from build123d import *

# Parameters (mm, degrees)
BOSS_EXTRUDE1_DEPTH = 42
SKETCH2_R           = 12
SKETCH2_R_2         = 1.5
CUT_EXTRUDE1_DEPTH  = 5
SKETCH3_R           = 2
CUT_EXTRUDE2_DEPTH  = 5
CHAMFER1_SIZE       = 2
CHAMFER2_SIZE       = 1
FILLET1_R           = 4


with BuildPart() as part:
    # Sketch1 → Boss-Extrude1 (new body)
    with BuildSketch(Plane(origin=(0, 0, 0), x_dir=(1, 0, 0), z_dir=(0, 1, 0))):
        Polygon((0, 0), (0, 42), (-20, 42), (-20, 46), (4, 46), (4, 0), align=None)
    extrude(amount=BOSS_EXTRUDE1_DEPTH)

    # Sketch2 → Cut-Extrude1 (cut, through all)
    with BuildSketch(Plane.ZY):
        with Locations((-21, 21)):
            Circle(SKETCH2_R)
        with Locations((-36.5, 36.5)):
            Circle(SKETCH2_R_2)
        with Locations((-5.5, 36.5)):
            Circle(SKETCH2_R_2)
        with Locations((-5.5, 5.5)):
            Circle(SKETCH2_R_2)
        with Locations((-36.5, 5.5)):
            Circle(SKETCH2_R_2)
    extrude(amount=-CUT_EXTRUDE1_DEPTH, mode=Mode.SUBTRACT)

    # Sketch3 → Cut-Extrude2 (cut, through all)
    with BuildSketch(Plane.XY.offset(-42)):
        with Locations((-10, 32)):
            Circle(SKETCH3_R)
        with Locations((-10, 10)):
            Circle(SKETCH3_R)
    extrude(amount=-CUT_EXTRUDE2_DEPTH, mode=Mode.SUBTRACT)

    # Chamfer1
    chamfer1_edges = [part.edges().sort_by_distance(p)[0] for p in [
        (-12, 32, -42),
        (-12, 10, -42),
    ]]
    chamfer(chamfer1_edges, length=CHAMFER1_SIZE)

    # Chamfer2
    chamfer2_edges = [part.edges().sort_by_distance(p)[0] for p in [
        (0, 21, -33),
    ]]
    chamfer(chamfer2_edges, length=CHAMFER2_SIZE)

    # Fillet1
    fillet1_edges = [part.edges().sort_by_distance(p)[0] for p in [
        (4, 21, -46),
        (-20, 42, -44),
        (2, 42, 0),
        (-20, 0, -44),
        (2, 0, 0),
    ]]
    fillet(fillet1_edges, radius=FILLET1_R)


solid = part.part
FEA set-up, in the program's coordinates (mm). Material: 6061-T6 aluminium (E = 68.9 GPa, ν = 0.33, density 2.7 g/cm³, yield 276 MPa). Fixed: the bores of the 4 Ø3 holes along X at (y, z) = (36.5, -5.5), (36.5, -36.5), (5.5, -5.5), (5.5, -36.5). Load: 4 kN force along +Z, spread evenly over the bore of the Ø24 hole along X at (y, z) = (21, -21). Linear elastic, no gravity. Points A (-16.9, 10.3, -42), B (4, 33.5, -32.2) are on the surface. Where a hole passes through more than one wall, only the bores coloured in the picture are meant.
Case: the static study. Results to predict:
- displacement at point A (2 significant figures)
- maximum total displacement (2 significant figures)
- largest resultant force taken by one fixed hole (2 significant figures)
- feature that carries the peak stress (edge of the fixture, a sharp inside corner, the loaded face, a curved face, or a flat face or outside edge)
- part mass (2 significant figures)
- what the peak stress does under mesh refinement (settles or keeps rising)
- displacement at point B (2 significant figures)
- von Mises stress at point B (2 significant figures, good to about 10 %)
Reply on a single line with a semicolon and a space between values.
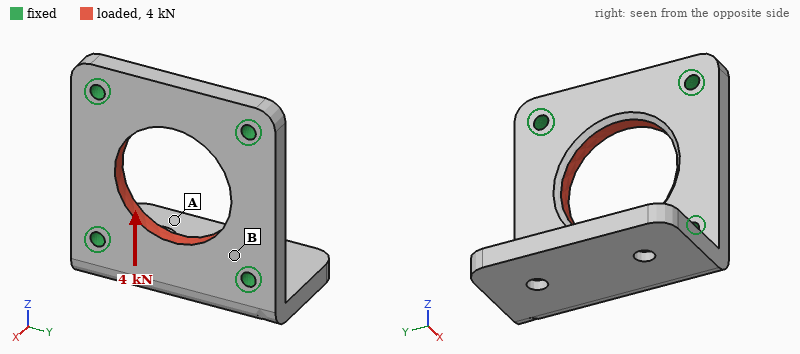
1.9 µm; 12 µm; 1.0 kN; edge of the fixture; 24 g; keeps rising; 2.1 µm; 24 MPa
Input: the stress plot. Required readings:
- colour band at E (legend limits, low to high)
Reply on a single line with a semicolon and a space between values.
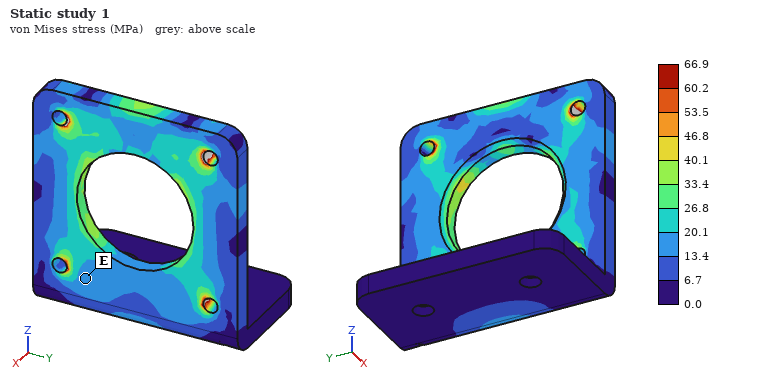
13.4 to 20.1 MPa
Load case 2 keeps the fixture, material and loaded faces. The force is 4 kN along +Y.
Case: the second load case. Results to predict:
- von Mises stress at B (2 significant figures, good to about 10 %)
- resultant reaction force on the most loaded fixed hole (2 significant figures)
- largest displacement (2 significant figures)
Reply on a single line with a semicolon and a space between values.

28 MPa; 1.0 kN; 11 µm
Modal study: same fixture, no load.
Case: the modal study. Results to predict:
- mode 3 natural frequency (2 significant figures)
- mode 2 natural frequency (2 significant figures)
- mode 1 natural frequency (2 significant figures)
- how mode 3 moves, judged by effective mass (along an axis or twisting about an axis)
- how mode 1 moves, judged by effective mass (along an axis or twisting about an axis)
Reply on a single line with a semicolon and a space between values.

14 kHz; 8100 Hz; 4200 Hz; along Y; along Z
